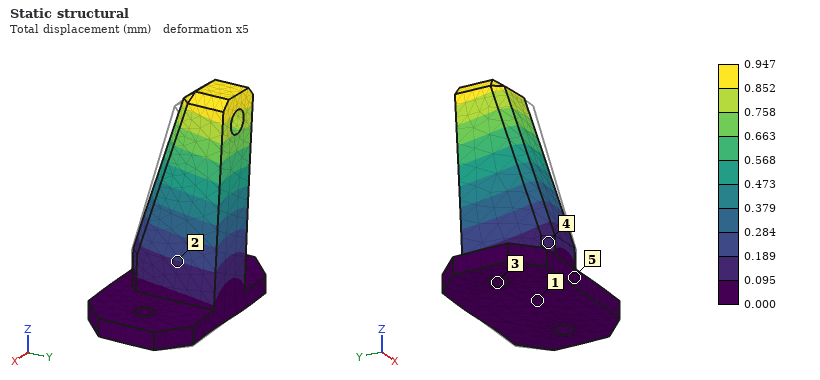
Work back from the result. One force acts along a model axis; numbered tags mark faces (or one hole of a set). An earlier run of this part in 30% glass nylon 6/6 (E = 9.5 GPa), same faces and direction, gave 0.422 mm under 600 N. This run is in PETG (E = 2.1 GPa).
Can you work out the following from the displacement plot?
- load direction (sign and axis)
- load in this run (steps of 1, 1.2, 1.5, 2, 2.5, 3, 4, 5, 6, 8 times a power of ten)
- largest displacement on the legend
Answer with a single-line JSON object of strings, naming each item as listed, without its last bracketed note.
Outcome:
{"load direction": "-X", "load in this run": "300 N", "largest displacement on the legend": "0.947 mm"}
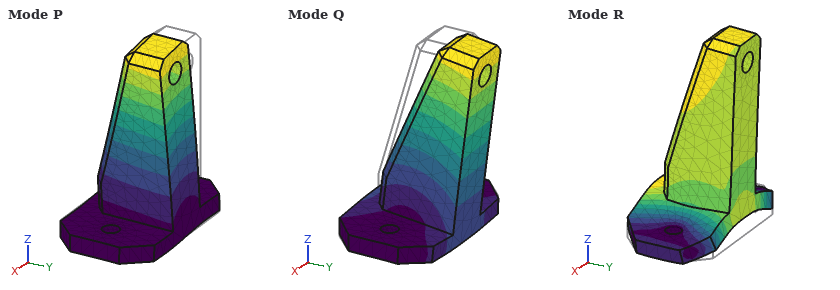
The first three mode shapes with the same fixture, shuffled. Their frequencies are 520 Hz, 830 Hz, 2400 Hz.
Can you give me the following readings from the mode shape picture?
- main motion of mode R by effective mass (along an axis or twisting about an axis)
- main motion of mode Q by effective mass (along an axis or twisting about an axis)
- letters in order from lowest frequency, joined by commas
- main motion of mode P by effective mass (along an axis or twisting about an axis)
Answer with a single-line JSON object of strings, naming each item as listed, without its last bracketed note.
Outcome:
{"main motion of mode R by effective mass": "along Z", "main motion of mode Q by effective mass": "along Y", "letters in order from lowest frequency, joined by commas": "Q, P, R", "main motion of mode P by effective mass": "along X"}
